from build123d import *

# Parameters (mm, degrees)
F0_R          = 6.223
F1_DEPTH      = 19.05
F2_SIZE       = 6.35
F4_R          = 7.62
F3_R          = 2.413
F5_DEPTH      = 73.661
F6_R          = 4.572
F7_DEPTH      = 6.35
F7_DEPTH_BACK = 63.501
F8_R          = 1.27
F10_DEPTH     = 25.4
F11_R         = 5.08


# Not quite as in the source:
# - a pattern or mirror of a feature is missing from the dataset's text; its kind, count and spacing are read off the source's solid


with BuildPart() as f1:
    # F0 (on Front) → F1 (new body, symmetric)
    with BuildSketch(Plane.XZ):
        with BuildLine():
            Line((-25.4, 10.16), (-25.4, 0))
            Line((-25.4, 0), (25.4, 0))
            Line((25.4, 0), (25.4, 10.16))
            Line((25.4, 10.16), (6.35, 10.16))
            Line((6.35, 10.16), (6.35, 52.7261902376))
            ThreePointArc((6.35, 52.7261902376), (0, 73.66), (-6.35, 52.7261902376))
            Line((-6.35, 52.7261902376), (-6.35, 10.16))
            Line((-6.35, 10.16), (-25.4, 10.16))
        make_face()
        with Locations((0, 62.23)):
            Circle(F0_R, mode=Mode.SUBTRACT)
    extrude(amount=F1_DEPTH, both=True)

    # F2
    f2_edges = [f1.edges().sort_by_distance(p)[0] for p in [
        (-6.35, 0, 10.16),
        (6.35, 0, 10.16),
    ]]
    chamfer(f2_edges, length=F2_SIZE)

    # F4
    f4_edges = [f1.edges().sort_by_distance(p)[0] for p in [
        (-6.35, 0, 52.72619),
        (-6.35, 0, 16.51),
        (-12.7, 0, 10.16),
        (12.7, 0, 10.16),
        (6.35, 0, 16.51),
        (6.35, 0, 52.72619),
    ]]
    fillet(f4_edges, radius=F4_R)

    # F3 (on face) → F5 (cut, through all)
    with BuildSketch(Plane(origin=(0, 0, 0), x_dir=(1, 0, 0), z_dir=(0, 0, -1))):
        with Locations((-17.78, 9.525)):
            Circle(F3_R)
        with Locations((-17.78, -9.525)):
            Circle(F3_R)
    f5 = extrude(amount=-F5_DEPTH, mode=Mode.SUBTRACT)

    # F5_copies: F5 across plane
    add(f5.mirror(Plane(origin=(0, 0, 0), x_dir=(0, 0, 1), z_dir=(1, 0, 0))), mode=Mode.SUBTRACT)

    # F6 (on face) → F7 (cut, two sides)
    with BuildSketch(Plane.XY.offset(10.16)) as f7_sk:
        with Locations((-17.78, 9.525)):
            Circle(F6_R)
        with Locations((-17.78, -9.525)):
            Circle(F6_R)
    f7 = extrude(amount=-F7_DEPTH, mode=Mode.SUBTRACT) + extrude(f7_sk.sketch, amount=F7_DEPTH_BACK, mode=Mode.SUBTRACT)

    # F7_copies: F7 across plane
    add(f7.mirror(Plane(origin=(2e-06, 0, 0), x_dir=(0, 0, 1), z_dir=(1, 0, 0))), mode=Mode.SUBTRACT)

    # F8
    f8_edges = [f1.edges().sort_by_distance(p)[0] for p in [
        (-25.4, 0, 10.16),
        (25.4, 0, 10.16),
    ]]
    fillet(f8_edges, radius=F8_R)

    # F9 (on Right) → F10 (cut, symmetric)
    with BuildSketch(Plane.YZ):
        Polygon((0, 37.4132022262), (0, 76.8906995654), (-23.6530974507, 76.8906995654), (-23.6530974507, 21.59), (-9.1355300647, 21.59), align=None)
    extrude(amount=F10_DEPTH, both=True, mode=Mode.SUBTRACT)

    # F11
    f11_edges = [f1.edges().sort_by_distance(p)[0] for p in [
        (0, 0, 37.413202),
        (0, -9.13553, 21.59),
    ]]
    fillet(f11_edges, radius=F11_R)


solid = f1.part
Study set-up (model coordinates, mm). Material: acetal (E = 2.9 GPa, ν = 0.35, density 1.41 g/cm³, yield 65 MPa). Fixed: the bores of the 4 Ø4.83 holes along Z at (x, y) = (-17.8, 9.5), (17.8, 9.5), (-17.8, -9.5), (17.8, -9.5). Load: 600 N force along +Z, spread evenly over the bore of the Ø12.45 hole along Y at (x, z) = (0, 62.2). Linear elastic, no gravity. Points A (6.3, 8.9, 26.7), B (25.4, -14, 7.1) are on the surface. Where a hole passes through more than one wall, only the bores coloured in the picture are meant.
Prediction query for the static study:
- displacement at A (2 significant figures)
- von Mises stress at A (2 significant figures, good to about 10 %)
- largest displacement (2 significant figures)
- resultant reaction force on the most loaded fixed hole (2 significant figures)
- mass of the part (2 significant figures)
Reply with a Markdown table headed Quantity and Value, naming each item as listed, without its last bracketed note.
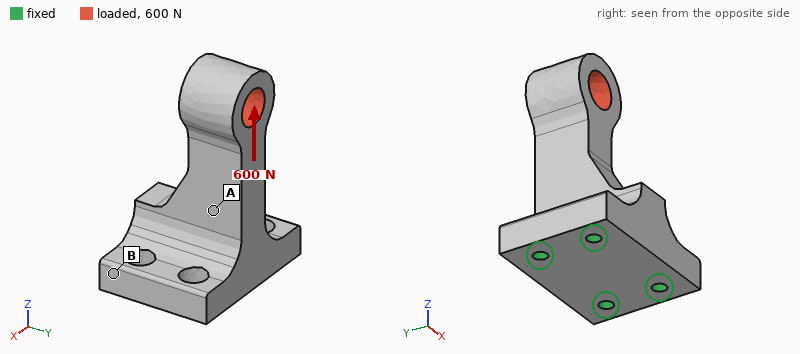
| Quantity | Value |
|---|---|
| displacement at A | 0.064 mm |
| von Mises stress at A | 2.3 MPa |
| largest displacement | 0.20 mm |
| resultant reaction force on the most loaded fixed hole | 320 N |
| mass of the part | 54 g |
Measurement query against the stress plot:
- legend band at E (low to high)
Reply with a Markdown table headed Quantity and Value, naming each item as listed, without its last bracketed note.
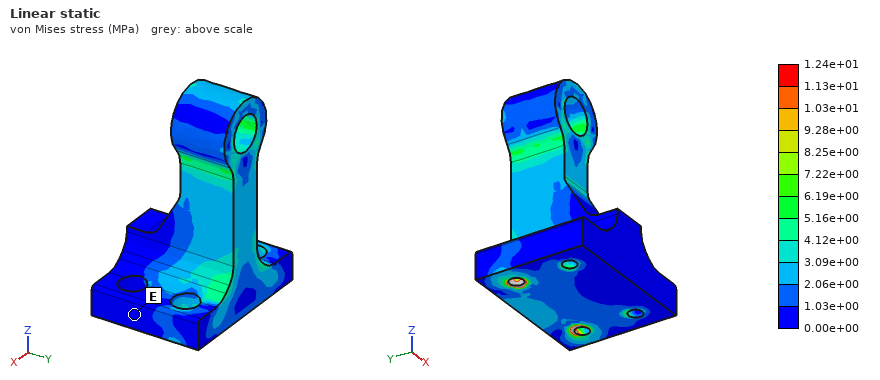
| Quantity | Value |
|---|---|
| legend band at E | 0.00e+00 to 1.03e+00 MPa |
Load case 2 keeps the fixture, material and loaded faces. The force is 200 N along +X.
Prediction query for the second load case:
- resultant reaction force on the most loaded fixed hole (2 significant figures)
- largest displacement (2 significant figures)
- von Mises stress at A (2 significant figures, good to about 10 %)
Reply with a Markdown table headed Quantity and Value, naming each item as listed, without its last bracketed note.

| Quantity | Value |
|---|---|
| resultant reaction force on the most loaded fixed hole | 220 N |
| largest displacement | 1.1 mm |
| von Mises stress at A | 11 MPa |
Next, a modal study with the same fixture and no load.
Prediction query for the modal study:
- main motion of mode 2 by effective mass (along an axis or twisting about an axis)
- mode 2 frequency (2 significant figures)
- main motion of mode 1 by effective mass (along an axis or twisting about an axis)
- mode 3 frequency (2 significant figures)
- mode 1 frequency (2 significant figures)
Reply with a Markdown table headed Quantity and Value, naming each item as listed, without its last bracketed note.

| Quantity | Value |
|---|---|
| main motion of mode 2 by effective mass | along Y |
| mode 2 frequency | 1000 Hz |
| main motion of mode 1 by effective mass | along X |
| mode 3 frequency | 2900 Hz |
| mode 1 frequency | 800 Hz |
